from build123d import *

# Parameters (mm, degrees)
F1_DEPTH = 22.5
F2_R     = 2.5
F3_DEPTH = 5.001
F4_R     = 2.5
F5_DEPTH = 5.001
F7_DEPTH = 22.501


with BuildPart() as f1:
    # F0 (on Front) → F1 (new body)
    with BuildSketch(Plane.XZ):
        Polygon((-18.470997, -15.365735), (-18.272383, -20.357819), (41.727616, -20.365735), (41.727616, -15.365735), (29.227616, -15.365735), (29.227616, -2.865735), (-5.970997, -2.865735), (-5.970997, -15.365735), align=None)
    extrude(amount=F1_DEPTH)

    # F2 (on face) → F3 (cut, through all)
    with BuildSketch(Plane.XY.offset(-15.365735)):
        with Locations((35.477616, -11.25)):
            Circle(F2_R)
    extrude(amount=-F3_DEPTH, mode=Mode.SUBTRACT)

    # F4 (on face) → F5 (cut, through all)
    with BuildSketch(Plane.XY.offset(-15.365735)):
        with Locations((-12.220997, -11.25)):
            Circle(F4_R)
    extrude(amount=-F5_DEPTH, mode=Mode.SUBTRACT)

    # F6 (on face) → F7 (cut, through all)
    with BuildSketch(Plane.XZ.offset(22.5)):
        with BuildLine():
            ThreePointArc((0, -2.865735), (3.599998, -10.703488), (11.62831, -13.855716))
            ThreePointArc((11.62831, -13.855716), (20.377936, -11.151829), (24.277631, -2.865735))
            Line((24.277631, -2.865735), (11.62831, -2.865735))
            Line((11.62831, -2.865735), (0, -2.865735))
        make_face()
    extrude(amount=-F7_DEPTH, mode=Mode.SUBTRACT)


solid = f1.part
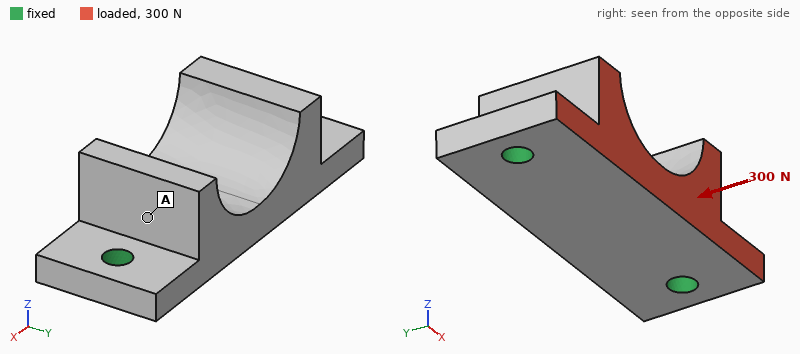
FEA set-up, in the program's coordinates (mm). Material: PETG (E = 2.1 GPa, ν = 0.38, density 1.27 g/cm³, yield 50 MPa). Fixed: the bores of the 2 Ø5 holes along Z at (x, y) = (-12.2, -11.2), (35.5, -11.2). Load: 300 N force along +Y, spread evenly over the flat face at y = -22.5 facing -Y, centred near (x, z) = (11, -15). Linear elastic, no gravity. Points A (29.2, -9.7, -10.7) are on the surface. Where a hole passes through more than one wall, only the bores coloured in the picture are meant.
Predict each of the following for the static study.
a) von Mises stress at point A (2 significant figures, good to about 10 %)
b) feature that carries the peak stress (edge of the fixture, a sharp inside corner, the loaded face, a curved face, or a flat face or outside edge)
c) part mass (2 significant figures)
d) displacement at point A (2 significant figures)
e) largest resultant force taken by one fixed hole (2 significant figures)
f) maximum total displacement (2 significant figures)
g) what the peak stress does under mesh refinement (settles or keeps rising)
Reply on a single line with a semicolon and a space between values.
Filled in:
1.2 MPa; edge of the fixture; 15 g; 0.052 mm; 150 N; 0.11 mm; keeps rising
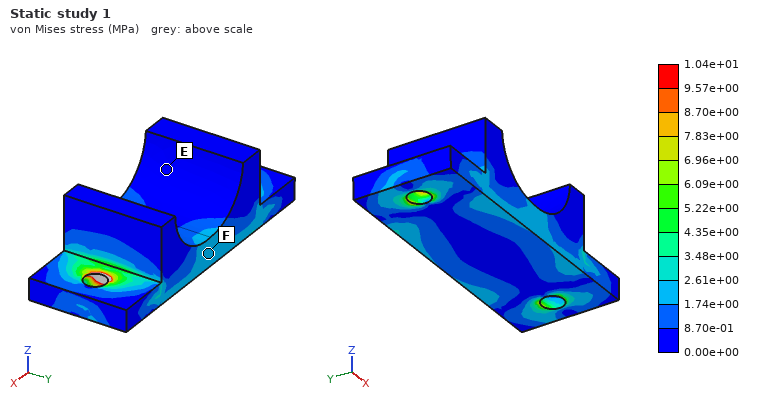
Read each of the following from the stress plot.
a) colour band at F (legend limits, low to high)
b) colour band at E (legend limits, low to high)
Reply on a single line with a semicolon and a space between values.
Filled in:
1.74e+00 to 2.61e+00 MPa; 0.00e+00 to 8.70e-01 MPa
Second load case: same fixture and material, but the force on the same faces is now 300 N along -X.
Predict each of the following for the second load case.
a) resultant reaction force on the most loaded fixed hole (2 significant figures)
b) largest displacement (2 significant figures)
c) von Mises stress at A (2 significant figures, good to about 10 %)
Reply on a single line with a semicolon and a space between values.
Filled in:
170 N; 42 µm; 0.73 MPa
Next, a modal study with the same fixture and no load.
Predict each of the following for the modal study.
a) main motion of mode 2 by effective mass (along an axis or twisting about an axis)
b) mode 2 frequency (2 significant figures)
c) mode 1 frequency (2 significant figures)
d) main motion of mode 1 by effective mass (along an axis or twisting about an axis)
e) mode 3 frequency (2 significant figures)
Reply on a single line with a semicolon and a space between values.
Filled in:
along Z; 2400 Hz; 2300 Hz; along Y; 4500 Hz
